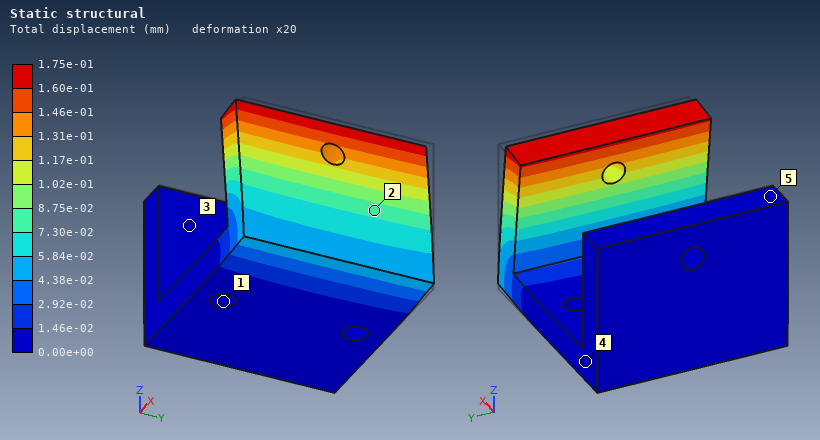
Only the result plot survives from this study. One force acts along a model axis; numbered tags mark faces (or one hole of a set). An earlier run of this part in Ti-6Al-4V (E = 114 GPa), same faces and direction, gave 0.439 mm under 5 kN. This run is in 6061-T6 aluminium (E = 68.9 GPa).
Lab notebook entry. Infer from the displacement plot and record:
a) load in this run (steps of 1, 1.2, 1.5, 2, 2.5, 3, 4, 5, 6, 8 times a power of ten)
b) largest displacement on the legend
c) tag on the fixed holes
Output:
1.2 kN
1.75e-01 mm
1
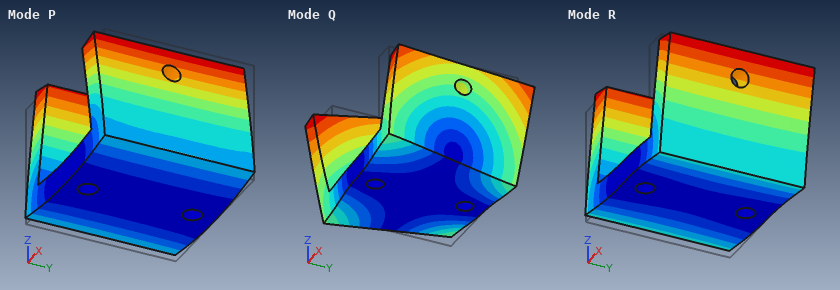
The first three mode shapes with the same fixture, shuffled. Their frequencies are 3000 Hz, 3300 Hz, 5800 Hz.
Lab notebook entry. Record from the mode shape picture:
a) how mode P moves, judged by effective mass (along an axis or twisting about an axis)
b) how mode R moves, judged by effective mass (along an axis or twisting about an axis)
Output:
along Z
along X
